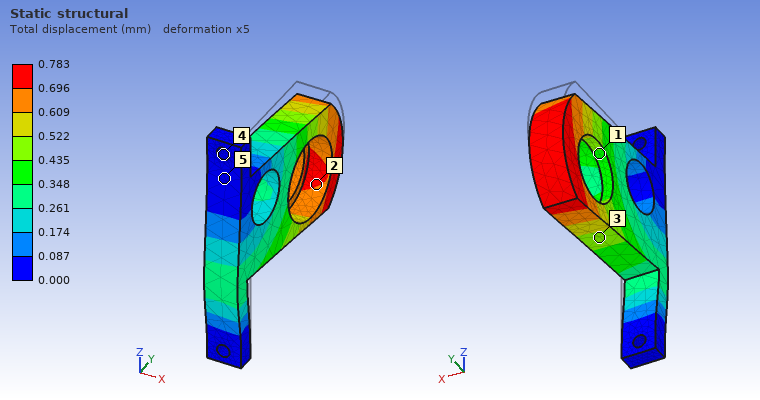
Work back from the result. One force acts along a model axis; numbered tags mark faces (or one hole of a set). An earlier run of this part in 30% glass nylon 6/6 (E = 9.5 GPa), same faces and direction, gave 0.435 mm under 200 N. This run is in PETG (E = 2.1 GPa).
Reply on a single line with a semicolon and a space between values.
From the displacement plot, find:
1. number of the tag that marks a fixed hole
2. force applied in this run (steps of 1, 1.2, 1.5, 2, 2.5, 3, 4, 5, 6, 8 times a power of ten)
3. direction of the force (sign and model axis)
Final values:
4; 80 N; -Z
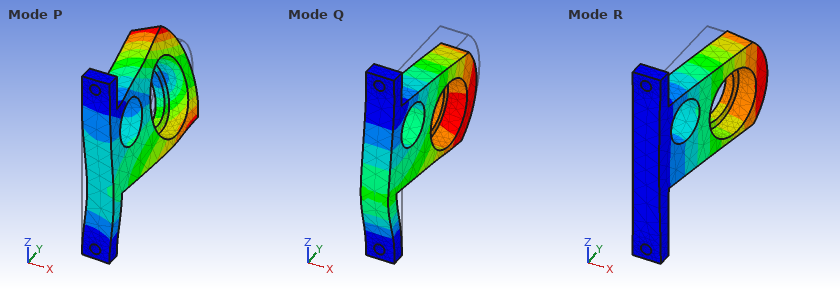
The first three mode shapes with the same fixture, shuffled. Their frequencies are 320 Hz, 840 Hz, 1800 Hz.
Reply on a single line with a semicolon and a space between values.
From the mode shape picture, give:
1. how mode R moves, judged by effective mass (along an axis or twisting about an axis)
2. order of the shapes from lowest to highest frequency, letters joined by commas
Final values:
along X; R, Q, P
